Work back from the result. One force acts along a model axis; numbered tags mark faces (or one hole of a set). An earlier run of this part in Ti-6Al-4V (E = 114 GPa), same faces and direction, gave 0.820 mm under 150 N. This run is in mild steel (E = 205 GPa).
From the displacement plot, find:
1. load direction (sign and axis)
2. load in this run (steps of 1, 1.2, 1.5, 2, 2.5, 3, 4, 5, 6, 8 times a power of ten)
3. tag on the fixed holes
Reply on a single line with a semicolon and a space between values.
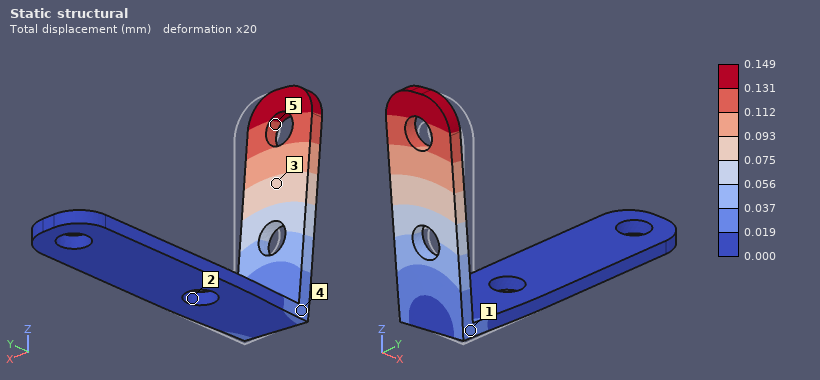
-X; 50 N; 2
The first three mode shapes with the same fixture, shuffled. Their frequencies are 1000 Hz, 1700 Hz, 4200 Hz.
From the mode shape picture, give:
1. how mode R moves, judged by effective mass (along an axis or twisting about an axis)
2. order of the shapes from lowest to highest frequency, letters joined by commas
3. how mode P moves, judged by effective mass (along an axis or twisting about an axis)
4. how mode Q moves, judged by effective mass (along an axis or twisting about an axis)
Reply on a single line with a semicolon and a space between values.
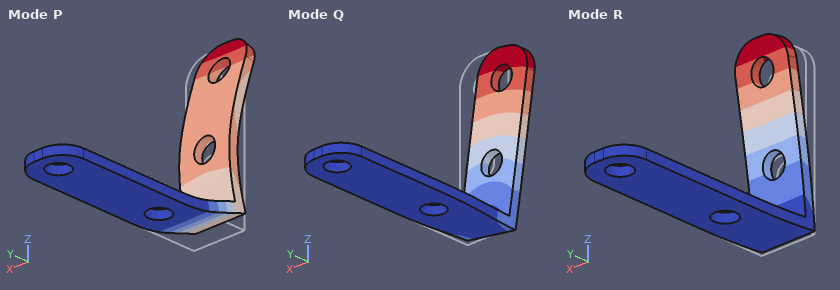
along Y; R, Q, P; along Z; along X
